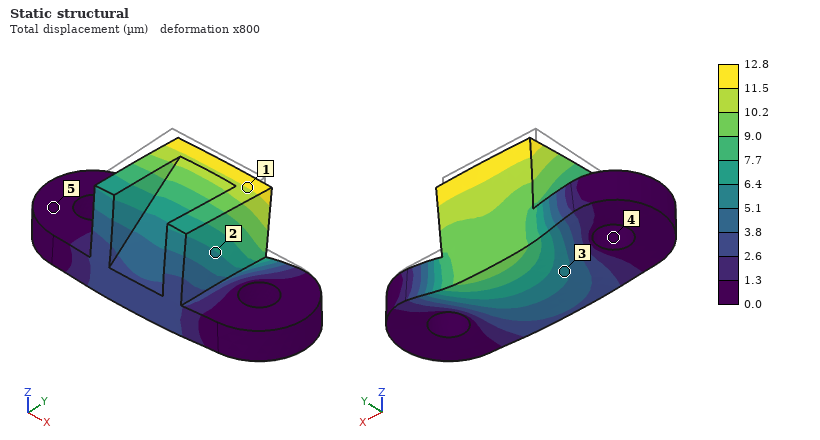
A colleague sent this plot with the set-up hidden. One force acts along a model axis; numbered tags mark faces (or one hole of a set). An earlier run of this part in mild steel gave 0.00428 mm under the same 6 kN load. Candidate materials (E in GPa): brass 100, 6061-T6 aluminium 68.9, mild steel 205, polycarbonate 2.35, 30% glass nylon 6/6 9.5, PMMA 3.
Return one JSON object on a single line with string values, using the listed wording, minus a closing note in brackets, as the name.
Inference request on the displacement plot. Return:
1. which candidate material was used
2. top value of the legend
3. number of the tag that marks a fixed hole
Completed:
{"which candidate material was used": "6061-T6 aluminium", "top value of the legend": "12.8 µm", "number of the tag that marks a fixed hole": "4"}
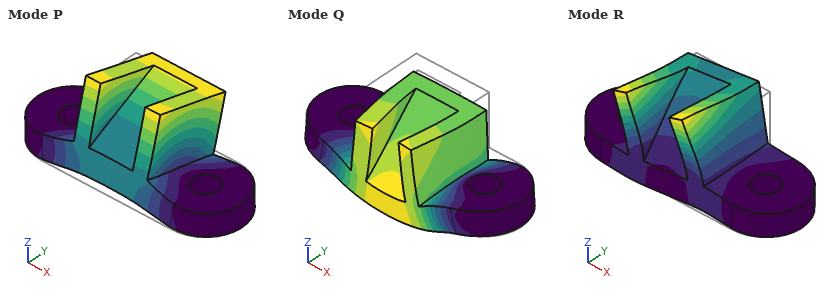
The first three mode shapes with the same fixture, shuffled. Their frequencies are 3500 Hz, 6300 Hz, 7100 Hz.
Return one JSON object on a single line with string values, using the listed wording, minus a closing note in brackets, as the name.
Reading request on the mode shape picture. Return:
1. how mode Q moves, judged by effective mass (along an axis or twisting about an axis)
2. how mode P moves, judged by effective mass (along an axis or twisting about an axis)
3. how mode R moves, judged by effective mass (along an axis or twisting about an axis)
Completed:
{"how mode Q moves, judged by effective mass": "along Z", "how mode P moves, judged by effective mass": "along Y", "how mode R moves, judged by effective mass": "along X"}
